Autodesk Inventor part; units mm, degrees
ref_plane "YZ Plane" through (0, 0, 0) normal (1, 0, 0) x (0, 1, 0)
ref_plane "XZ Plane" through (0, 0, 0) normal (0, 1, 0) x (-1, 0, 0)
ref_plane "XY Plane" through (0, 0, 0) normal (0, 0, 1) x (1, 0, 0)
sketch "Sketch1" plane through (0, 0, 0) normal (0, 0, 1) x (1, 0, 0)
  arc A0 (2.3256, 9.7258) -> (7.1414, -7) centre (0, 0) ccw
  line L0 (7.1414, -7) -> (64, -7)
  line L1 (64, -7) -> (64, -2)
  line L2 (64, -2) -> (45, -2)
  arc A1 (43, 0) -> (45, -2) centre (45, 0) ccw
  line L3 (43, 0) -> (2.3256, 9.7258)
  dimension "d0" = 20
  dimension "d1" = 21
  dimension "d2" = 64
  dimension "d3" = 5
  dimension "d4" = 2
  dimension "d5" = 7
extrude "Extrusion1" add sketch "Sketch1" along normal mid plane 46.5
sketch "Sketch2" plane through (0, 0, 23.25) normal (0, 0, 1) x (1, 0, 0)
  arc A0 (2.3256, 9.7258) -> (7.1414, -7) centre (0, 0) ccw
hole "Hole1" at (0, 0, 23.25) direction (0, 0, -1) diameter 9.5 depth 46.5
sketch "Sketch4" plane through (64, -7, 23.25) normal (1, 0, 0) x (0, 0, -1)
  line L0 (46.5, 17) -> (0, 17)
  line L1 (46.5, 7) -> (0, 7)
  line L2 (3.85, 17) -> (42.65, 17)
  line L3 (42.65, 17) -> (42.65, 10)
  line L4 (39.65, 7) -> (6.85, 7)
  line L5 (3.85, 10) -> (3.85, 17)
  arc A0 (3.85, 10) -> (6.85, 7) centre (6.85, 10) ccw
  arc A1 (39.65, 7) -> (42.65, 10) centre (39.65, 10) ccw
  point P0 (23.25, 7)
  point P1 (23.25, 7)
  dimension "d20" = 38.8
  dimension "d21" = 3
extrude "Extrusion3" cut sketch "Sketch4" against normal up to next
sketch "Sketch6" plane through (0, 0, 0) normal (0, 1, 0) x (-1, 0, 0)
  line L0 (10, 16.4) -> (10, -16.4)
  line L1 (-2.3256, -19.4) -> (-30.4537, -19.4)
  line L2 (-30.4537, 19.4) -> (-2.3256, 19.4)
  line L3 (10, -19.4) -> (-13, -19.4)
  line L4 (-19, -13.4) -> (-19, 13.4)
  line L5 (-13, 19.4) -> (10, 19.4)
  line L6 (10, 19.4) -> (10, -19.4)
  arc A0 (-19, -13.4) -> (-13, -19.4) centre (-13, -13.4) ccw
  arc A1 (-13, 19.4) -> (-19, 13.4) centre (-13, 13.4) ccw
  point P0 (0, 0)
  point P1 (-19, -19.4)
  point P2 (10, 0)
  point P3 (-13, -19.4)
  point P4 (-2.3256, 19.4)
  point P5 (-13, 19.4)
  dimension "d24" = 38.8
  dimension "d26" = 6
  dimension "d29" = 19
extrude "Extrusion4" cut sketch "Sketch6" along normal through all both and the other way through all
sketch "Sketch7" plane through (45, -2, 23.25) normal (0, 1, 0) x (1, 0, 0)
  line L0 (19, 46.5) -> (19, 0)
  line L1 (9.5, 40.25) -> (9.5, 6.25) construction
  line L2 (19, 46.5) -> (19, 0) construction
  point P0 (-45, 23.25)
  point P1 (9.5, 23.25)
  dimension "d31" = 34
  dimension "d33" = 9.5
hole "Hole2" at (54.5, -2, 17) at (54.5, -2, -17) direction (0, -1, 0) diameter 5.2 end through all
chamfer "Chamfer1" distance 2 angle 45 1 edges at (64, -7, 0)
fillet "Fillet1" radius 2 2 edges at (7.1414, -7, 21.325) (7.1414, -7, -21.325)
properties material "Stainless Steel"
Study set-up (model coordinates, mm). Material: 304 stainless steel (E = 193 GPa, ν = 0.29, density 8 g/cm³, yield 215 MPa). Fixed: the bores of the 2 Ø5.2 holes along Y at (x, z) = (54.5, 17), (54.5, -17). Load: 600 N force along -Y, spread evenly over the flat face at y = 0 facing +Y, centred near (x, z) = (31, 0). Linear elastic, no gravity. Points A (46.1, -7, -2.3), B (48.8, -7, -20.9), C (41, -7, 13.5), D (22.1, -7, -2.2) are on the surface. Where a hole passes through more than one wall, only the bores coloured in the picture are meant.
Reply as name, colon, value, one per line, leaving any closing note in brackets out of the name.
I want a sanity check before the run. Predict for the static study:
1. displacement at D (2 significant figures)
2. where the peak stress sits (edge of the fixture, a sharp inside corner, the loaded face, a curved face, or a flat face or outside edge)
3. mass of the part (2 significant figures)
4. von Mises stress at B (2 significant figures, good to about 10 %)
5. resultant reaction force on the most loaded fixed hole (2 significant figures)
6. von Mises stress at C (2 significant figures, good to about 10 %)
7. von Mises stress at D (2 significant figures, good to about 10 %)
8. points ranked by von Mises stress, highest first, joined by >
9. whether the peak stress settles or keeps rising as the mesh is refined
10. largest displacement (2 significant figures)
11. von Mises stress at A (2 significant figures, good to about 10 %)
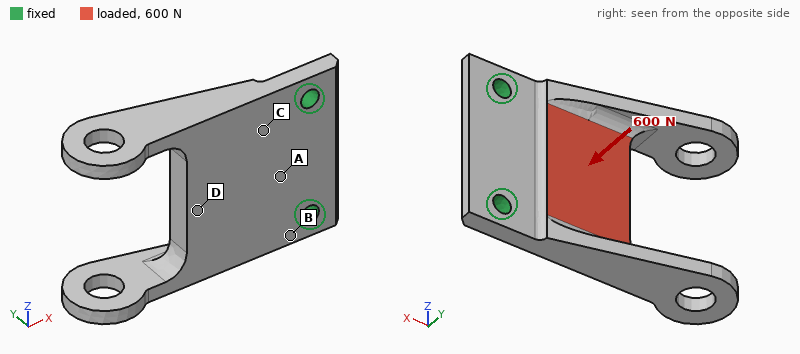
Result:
displacement at D: 44 µm
where the peak stress sits: edge of the fixture
mass of the part: 130 g
von Mises stress at B: 64 MPa
resultant reaction force on the most loaded fixed hole: 300 N
von Mises stress at C: 20 MPa
von Mises stress at D: 9.9 MPa
points ranked by von Mises stress, highest first, joined by >: B > A > C > D
whether the peak stress settles or keeps rising as the mesh is refined: keeps rising
largest displacement: 93 µm
von Mises stress at A: 34 MPa
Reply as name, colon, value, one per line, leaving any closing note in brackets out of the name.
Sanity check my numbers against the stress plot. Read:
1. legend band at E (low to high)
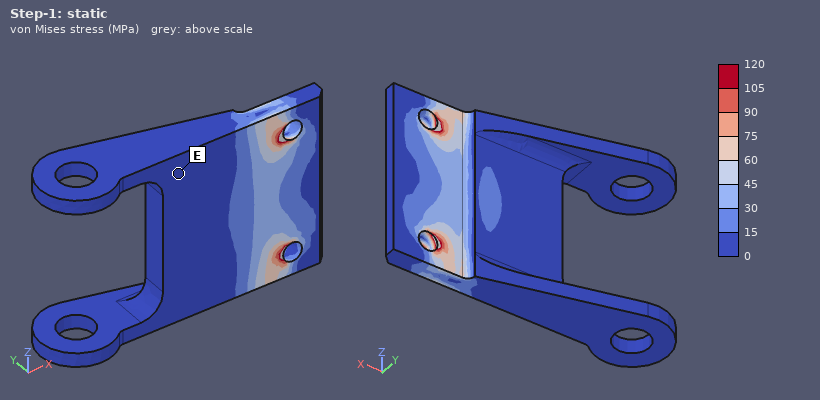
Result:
legend band at E: 0 to 15 MPa
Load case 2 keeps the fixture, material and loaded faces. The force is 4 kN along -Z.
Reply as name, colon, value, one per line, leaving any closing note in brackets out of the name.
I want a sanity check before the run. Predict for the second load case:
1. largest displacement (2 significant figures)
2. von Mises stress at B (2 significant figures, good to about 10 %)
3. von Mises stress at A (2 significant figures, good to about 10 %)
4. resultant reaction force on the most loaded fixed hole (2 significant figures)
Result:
largest displacement: 33 µm
von Mises stress at B: 55 MPa
von Mises stress at A: 17 MPa
resultant reaction force on the most loaded fixed hole: 3.3 kN
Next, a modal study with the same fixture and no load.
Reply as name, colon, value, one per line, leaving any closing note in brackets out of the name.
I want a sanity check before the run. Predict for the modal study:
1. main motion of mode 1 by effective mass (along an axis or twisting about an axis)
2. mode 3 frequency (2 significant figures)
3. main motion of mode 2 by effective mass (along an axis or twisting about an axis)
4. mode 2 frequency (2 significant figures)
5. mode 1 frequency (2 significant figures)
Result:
main motion of mode 1 by effective mass: along Y
mode 3 frequency: 3600 Hz
main motion of mode 2 by effective mass: twisting about X
mode 2 frequency: 2900 Hz
mode 1 frequency: 1500 Hz
